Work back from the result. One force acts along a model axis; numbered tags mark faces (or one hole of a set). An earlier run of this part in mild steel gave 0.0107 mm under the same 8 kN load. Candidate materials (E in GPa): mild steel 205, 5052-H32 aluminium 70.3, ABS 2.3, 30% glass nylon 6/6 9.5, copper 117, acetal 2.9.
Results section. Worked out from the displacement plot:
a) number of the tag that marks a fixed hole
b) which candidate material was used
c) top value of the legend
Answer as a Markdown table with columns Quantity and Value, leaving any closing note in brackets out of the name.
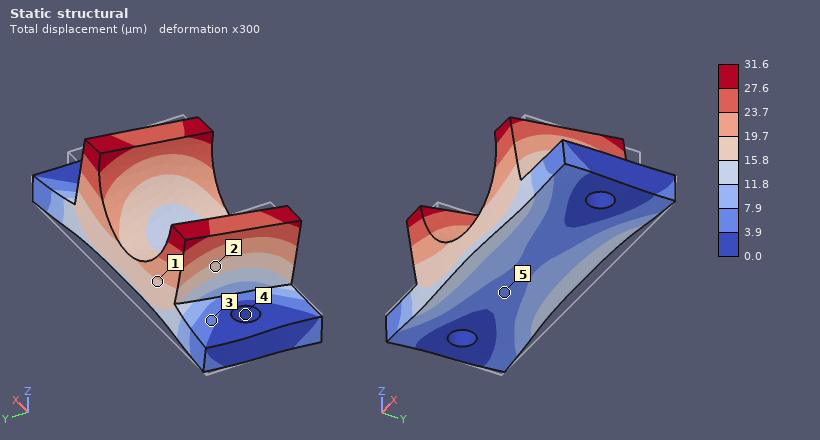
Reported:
| Quantity | Value |
|---|---|
| number of the tag that marks a fixed hole | 4 |
| which candidate material was used | 5052-H32 aluminium |
| top value of the legend | 31.6 µm |
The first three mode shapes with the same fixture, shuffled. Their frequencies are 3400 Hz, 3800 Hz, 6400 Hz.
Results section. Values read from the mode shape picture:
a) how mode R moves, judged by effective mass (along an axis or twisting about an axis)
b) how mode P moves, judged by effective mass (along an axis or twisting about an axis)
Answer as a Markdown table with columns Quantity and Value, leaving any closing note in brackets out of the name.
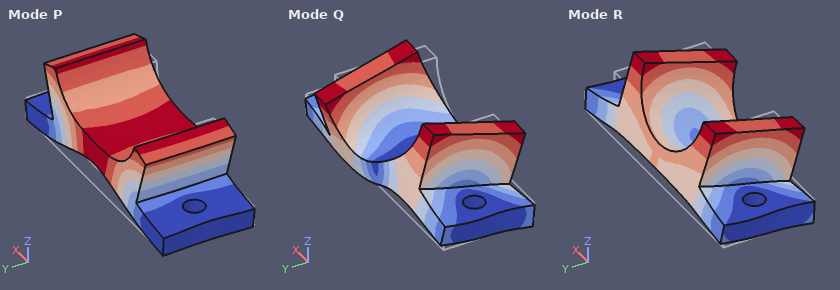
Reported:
| Quantity | Value |
|---|---|
| how mode R moves, judged by effective mass | along Y |
| how mode P moves, judged by effective mass | along Z |
